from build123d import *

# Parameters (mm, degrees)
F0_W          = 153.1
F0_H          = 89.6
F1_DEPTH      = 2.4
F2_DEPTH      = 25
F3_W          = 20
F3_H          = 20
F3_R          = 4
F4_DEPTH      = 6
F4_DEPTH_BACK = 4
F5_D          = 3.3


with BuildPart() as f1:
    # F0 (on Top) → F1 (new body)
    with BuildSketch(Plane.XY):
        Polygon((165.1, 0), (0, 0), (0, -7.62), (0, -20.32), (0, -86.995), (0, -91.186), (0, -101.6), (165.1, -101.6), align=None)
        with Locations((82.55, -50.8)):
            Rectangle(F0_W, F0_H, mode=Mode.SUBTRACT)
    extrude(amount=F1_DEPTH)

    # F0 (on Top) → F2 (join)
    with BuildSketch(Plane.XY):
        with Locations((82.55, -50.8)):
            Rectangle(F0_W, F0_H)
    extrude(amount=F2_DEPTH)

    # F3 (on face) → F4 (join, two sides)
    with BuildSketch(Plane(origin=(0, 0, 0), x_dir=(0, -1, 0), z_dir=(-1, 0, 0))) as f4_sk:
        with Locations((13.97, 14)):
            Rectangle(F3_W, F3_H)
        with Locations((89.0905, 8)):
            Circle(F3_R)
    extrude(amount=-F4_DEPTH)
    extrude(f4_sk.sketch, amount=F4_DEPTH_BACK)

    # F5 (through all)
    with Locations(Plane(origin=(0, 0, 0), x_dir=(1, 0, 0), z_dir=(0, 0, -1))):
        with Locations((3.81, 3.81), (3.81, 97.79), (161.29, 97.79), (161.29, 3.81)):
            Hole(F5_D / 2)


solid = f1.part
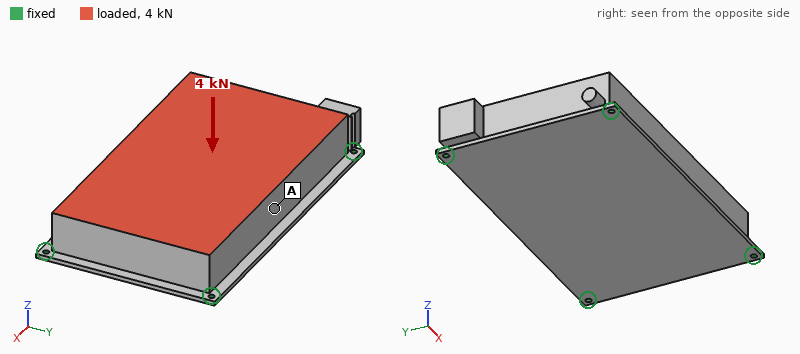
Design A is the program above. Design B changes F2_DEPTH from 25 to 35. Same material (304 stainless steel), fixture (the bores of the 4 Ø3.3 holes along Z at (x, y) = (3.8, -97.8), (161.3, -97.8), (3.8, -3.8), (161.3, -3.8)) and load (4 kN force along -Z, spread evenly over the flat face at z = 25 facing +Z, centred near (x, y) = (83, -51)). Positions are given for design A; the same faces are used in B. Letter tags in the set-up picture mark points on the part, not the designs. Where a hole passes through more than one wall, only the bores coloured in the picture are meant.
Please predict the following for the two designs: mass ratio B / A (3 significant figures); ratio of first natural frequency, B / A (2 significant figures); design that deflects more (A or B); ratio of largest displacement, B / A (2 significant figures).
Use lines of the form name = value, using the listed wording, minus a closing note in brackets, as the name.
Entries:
mass ratio B / A = 1.39
ratio of first natural frequency, B / A = 0.95
design that deflects more = A
ratio of largest displacement, B / A = 0.74
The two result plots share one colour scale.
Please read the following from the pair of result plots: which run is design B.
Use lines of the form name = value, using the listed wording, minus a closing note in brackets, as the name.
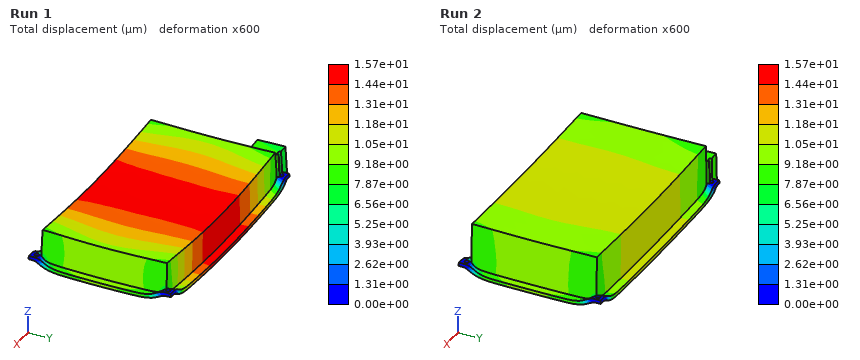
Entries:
which run is design B = Run 2
